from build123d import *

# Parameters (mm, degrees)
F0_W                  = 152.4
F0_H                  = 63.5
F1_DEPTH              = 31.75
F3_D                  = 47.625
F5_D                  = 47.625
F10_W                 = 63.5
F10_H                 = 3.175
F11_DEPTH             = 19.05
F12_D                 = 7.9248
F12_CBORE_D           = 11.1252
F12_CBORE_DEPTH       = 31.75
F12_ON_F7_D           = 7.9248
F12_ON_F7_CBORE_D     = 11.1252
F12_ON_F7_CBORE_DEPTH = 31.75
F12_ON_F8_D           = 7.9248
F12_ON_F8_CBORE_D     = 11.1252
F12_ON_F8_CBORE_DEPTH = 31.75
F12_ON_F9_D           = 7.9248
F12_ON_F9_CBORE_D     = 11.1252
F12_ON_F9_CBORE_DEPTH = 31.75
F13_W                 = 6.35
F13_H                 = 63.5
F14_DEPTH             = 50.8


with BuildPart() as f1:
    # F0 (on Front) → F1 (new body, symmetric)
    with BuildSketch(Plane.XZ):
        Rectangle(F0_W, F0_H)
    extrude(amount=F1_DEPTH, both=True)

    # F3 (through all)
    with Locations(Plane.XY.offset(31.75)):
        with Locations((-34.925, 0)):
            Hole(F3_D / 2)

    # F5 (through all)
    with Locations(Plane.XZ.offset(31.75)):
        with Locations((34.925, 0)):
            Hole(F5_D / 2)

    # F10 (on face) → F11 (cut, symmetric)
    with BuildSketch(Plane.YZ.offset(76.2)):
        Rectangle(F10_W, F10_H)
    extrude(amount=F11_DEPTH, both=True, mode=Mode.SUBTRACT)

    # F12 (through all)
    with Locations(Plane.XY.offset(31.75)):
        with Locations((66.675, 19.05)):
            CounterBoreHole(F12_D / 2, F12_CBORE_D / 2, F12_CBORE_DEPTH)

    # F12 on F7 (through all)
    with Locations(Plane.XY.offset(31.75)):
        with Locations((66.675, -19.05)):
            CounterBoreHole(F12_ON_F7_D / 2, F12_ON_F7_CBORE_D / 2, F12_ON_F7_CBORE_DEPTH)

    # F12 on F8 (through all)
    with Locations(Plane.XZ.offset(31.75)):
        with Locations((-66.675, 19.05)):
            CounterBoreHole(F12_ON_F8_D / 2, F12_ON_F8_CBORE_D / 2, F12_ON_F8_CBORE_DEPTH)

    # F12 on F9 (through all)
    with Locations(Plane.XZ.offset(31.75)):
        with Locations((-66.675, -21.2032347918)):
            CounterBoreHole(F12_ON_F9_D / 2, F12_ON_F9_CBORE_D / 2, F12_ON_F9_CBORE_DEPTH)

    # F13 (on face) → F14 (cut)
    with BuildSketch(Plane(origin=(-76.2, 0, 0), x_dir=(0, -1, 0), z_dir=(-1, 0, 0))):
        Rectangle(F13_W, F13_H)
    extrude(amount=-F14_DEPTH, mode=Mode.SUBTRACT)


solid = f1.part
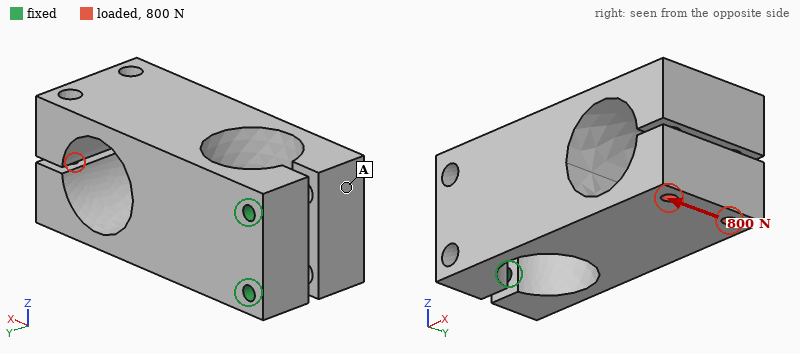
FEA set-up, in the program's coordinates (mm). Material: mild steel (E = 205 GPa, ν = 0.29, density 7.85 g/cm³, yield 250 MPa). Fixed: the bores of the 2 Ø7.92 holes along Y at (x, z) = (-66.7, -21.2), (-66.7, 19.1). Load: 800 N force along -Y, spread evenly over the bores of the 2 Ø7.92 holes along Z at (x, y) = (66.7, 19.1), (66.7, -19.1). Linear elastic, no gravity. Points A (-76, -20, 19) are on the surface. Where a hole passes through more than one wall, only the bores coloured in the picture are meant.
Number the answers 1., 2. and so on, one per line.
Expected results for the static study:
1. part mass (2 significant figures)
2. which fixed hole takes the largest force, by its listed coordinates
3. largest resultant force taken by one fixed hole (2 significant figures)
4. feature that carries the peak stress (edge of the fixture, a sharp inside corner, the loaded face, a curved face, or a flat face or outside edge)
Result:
1. 2.8 kg
2. (-66.7, -21.2)
3. 640 N
4. a flat face or outside edge
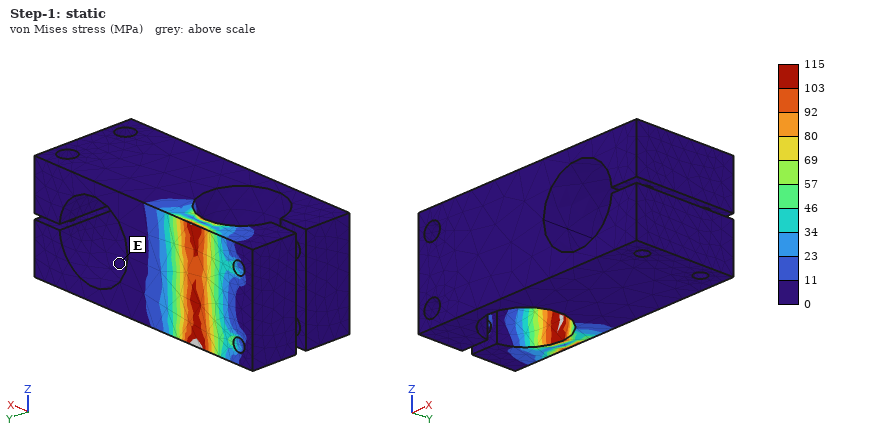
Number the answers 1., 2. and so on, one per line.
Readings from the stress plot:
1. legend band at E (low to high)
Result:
1. 0 to 11 MPa
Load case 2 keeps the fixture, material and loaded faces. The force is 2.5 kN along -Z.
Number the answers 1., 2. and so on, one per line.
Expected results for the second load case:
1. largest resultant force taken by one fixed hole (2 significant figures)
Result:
1. 7.6 kN
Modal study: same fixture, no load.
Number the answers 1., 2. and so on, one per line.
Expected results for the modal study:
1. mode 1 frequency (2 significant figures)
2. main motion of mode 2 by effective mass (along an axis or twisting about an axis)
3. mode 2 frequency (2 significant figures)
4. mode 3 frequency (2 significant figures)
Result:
1. 220 Hz
2. along Z
3. 650 Hz
4. 1000 Hz
